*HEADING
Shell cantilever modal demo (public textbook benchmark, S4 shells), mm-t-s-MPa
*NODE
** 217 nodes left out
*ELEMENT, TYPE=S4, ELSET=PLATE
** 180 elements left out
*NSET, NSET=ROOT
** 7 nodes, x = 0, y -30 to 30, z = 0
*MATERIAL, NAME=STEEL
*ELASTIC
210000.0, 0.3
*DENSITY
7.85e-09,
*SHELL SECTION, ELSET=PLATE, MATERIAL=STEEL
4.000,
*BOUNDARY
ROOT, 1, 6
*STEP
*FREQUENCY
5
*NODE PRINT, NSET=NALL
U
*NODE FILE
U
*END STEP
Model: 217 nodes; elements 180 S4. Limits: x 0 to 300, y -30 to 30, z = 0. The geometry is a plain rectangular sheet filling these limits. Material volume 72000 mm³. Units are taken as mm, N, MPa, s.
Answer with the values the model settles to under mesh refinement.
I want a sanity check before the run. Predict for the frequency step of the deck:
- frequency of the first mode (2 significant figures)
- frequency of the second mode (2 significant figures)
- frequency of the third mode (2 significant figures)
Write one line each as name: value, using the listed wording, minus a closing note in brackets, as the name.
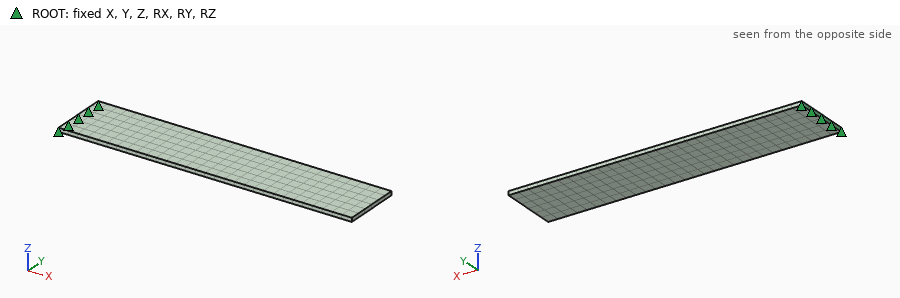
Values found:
frequency of the first mode: 38 Hz
frequency of the second mode: 240 Hz
frequency of the third mode: 370 Hz
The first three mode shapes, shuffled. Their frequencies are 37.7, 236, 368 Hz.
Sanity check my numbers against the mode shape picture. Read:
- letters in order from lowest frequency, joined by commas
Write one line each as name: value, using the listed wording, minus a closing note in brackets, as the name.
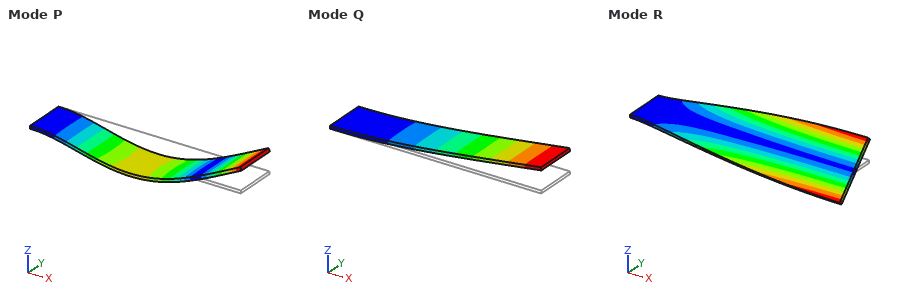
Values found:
letters in order from lowest frequency, joined by commas: Q, P, R
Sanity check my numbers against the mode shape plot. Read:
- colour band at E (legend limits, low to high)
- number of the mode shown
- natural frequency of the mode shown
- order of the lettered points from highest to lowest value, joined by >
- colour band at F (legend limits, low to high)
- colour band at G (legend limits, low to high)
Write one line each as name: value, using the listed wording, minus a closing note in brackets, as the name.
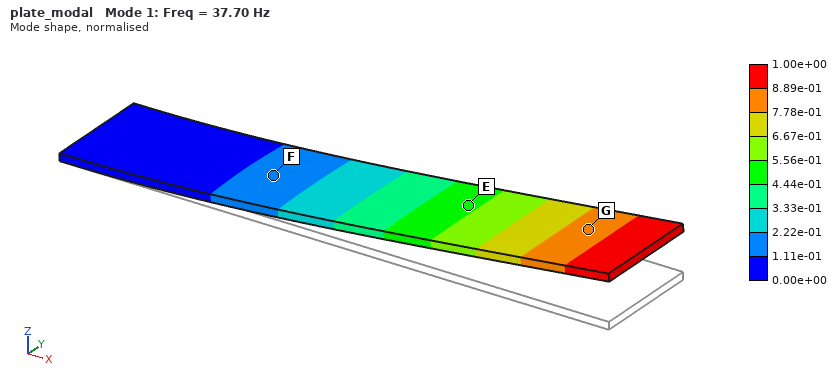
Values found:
colour band at E: 4.44e-01 to 5.56e-01
number of the mode shown: 1
natural frequency of the mode shown: 37.70 Hz
order of the lettered points from highest to lowest value, joined by >: G > E > F
colour band at F: 1.11e-01 to 2.22e-01
colour band at G: 7.78e-01 to 8.89e-01
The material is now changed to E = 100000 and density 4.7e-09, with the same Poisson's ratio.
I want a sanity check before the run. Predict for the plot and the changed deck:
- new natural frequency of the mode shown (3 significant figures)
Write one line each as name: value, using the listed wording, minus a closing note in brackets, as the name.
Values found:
new natural frequency of the mode shown: 33.6 Hz
